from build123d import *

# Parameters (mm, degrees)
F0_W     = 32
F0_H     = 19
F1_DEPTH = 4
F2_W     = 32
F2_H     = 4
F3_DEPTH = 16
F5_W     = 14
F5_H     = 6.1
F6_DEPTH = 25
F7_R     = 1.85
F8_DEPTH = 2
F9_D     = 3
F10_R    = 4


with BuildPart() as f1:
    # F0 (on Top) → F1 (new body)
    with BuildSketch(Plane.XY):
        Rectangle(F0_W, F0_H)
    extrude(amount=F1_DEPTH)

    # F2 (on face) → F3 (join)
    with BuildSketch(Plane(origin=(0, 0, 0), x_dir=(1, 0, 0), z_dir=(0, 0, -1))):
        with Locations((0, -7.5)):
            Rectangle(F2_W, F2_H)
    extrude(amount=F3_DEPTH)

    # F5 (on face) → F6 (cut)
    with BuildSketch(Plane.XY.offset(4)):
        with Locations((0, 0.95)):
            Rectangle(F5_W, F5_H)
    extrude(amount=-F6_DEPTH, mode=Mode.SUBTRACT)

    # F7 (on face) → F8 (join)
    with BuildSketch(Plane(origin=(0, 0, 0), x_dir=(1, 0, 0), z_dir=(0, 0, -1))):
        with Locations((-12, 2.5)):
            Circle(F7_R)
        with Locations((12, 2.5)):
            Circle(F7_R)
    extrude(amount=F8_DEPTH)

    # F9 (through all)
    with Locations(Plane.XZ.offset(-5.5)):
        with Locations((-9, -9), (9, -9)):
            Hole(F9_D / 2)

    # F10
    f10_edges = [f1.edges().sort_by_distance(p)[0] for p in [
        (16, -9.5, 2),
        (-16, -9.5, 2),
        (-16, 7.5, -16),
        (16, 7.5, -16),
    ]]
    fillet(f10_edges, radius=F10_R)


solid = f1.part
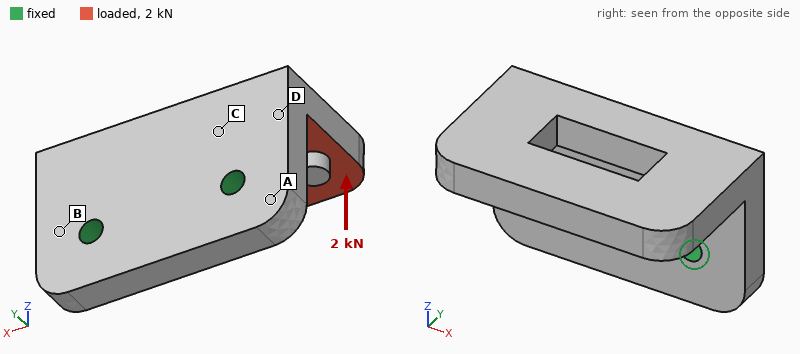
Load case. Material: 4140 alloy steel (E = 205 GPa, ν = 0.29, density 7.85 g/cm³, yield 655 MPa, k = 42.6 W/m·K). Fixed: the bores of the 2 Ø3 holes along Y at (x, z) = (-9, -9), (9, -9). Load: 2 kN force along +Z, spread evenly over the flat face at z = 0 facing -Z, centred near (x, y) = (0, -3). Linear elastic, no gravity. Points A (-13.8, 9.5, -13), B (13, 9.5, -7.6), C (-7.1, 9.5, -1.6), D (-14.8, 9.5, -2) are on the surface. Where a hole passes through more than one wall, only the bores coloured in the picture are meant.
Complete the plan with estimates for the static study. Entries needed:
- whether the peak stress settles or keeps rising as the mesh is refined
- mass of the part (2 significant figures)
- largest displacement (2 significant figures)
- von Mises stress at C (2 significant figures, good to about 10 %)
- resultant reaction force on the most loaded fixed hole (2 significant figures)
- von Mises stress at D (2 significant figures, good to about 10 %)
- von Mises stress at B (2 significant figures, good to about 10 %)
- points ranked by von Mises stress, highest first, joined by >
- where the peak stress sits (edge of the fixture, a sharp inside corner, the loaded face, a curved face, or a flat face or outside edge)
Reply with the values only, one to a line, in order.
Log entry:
keeps rising
32 g
0.19 mm
200 MPa
1.0 kN
260 MPa
150 MPa
D > C > B > A
edge of the fixture
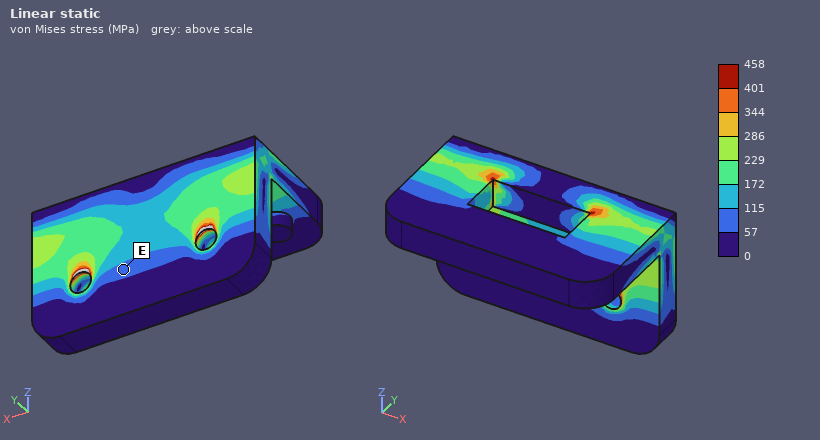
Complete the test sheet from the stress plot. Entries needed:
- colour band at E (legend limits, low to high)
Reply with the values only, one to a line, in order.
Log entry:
57 to 115 MPa
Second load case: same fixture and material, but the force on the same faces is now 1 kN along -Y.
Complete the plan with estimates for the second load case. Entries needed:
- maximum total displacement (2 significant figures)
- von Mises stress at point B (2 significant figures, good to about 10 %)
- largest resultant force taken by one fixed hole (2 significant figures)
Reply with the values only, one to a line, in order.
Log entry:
18 µm
56 MPa
500 N
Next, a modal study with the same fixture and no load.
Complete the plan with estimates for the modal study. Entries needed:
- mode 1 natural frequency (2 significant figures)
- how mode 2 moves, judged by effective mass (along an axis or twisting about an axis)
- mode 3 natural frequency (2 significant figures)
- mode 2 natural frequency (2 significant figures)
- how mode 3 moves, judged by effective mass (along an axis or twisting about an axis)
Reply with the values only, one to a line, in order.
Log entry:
5200 Hz
along X
13 kHz
8900 Hz
along Y
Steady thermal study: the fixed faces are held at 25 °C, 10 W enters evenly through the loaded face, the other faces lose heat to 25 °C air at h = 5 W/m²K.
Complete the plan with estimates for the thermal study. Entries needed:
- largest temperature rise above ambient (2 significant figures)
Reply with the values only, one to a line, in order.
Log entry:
54 K
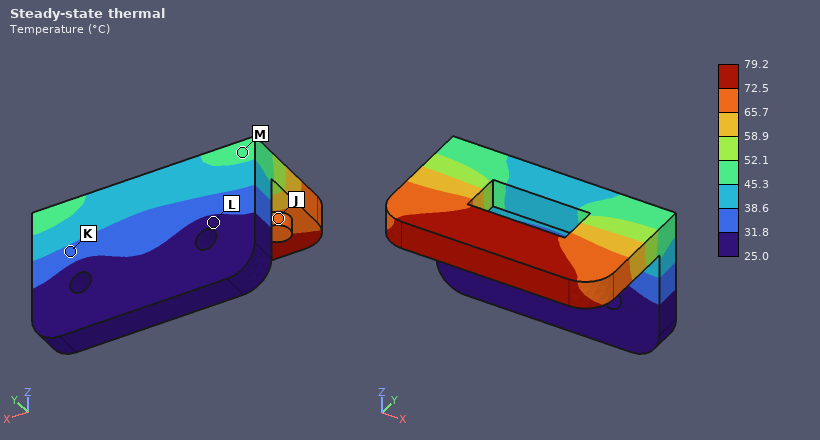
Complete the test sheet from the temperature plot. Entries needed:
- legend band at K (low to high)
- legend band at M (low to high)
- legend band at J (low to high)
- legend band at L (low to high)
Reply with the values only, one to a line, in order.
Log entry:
31.8 to 38.6 °C
45.3 to 52.1 °C
65.7 to 72.5 °C
25.0 to 31.8 °C
